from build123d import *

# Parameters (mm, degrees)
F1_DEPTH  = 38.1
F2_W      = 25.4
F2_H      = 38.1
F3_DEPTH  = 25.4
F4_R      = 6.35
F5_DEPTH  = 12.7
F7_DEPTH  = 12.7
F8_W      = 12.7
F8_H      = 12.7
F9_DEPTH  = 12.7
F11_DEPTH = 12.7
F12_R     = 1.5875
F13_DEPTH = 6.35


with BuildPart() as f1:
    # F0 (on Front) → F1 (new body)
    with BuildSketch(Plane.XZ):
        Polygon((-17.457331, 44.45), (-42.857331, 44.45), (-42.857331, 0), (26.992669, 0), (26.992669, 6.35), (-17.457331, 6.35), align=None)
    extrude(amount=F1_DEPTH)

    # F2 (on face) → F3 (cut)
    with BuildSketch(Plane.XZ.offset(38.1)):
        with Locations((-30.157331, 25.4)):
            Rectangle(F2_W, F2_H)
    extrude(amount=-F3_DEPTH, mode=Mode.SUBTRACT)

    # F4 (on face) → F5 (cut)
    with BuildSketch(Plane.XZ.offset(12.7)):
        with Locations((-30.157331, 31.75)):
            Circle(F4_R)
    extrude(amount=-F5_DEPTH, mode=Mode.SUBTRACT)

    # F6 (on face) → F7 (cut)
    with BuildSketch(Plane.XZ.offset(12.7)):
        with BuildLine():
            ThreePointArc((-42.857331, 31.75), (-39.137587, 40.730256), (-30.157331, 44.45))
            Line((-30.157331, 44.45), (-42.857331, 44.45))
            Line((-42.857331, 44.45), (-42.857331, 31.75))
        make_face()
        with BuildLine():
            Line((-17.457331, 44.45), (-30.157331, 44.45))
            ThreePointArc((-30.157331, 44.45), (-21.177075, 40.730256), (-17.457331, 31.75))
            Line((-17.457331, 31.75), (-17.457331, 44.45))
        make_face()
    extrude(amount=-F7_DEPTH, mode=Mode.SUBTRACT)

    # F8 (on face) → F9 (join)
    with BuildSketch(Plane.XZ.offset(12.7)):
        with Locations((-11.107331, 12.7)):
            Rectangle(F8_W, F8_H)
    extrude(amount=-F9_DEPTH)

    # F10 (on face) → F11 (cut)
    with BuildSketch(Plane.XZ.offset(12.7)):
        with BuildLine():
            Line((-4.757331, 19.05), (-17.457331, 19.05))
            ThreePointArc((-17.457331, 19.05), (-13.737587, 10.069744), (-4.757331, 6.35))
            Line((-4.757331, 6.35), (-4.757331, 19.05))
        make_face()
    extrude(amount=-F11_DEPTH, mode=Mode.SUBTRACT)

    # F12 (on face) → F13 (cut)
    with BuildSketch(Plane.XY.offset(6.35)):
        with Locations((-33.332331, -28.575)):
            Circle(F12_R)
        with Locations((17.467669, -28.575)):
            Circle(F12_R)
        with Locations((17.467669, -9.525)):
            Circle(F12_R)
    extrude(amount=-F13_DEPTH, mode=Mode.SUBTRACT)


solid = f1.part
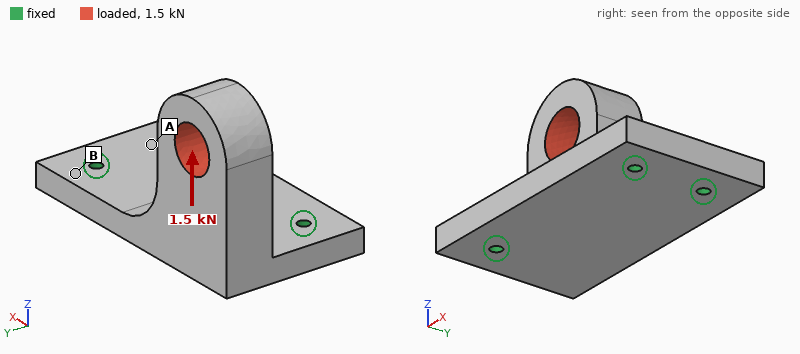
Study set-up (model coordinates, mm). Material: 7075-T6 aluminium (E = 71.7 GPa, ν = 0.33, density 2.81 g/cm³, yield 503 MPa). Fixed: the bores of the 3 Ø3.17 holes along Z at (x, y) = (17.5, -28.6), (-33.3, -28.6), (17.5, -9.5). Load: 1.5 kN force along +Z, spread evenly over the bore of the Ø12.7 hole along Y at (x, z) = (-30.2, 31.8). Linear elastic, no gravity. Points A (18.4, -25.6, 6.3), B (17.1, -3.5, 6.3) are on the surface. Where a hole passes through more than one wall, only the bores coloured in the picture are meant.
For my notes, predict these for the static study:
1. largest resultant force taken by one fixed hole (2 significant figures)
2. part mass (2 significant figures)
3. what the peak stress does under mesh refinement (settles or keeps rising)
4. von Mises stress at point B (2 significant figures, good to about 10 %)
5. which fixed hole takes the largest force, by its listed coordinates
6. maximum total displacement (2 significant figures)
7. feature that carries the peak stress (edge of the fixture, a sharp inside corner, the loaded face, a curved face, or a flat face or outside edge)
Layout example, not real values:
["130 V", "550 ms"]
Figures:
["1.3 kN", "76 g", "keeps rising", "34 MPa", "(-33.3, -28.6)", "0.26 mm", "edge of the fixture"]
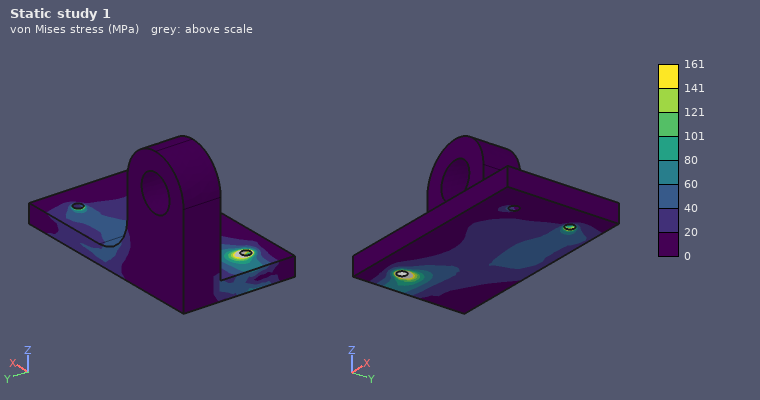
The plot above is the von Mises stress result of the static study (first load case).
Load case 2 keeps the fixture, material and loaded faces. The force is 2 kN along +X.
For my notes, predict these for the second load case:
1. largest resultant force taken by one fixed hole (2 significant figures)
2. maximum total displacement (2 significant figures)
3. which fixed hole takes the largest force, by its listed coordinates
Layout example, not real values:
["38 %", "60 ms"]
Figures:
["1.4 kN", "0.26 mm", "(-33.3, -28.6)"]
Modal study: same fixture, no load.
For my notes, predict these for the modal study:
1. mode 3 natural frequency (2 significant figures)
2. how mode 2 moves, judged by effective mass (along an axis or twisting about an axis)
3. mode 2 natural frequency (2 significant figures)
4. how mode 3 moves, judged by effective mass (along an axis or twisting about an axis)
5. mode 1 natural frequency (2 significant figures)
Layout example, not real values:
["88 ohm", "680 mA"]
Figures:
["6300 Hz", "along X", "4300 Hz", "along Z", "2100 Hz"]
